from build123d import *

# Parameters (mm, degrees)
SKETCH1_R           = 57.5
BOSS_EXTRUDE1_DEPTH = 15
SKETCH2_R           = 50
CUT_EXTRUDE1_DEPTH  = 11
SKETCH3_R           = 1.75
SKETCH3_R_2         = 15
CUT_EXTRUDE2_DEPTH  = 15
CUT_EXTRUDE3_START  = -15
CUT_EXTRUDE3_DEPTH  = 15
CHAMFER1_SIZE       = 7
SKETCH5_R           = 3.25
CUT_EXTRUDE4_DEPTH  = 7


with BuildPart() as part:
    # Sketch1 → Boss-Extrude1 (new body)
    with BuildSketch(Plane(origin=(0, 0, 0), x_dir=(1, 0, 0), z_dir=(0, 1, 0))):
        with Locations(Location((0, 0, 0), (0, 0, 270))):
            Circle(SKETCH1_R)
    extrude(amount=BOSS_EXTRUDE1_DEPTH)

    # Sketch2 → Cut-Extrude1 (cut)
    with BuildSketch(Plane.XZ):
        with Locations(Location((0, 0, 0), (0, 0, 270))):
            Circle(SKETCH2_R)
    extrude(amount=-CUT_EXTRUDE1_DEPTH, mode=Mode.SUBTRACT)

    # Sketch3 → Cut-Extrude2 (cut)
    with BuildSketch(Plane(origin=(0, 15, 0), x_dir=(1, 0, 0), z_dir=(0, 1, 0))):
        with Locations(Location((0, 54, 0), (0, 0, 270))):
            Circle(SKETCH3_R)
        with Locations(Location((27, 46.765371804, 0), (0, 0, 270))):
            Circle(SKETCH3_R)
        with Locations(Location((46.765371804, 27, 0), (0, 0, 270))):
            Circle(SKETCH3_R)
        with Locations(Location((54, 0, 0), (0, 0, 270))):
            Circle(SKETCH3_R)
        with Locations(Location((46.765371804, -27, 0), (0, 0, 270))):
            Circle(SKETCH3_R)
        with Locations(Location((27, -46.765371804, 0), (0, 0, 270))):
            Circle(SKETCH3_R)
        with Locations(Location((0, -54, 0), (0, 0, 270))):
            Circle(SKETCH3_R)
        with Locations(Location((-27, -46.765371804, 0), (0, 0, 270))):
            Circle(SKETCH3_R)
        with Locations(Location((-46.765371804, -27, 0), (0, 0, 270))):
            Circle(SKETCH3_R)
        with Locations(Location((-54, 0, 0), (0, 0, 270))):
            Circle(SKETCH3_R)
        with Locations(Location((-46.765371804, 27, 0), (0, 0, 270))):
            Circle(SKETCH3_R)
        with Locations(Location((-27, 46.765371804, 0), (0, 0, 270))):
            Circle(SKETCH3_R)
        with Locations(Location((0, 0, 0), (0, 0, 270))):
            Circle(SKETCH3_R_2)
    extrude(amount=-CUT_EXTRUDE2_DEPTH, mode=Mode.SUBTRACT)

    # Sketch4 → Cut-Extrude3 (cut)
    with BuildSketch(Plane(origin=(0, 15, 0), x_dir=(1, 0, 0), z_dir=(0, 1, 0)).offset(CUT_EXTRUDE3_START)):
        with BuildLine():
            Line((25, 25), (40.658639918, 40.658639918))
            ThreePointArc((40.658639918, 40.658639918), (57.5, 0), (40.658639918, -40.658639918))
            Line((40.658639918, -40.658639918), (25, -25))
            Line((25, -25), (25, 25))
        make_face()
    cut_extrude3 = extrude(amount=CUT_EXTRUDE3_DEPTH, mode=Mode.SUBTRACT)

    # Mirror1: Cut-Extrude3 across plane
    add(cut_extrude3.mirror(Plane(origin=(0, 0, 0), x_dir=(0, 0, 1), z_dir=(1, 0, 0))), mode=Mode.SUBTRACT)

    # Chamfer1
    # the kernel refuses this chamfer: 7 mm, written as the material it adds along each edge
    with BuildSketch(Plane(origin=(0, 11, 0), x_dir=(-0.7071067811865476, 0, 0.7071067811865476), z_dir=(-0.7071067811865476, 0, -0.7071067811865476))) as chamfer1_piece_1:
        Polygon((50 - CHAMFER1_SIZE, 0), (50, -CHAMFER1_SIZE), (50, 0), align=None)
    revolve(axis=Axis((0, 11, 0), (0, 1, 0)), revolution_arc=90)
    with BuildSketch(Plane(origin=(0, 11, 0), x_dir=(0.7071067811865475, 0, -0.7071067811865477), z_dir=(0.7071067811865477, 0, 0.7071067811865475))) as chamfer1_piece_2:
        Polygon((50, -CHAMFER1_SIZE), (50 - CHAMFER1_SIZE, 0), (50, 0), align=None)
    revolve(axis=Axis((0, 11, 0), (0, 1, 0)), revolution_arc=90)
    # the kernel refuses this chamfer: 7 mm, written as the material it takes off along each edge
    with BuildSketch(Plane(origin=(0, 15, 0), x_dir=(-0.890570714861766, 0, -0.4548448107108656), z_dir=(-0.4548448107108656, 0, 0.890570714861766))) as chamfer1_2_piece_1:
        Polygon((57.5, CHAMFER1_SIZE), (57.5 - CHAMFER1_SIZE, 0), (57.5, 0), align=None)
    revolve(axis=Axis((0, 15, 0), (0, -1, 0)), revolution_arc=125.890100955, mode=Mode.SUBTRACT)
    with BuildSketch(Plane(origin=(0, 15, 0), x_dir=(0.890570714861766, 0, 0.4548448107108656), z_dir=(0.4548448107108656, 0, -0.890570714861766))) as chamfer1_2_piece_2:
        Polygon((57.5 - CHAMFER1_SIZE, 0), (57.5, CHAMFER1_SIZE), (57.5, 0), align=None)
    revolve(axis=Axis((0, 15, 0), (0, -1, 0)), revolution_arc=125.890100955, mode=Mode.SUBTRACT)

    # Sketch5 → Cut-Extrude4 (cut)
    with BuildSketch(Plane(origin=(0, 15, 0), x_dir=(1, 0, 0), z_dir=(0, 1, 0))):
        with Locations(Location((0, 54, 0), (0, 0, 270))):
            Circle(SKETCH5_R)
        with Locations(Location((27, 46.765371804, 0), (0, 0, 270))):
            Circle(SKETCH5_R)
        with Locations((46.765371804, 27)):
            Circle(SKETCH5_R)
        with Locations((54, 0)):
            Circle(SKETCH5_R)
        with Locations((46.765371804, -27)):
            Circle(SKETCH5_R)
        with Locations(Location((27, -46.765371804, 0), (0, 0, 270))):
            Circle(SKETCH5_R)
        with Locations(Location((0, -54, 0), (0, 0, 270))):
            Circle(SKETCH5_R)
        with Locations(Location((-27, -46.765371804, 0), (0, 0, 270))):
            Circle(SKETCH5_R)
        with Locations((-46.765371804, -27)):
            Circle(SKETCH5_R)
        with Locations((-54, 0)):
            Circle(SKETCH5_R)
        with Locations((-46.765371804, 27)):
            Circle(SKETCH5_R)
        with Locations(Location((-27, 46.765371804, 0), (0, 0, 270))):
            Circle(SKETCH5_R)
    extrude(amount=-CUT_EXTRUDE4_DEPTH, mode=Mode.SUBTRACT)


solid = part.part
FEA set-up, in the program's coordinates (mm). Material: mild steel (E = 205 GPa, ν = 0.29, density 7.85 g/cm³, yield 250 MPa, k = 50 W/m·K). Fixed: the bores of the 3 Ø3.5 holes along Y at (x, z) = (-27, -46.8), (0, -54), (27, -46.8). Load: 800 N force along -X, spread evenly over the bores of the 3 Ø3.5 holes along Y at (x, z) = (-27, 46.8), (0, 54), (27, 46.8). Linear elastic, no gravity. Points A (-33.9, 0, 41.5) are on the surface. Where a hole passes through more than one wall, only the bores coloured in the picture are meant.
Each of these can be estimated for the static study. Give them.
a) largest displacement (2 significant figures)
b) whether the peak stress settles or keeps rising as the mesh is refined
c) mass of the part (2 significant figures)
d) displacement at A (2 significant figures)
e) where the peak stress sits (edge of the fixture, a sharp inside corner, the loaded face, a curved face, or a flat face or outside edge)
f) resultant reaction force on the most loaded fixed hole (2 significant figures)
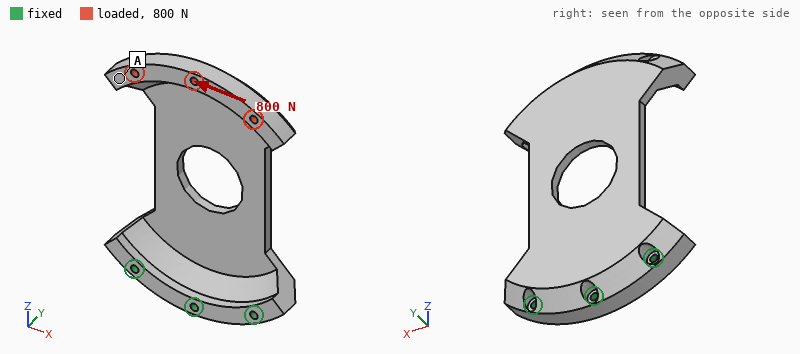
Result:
0.32 mm
keeps rising
280 g
0.28 mm
edge of the fixture
1.4 kN
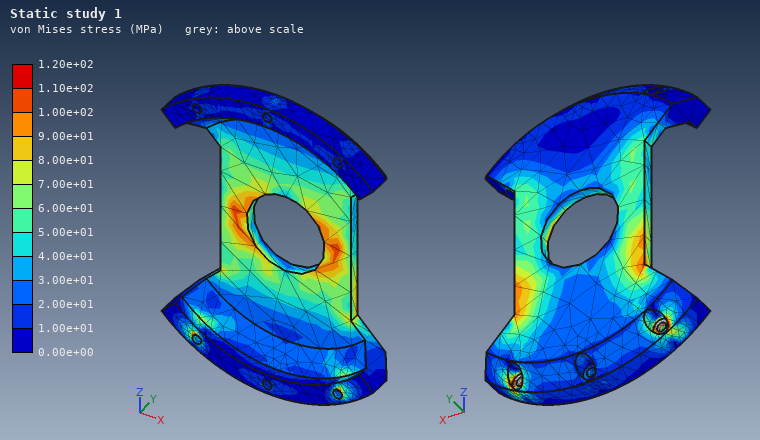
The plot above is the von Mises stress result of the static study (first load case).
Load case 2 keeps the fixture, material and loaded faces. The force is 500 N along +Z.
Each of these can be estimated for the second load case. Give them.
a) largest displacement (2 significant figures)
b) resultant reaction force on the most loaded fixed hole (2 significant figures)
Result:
0.55 mm
200 N
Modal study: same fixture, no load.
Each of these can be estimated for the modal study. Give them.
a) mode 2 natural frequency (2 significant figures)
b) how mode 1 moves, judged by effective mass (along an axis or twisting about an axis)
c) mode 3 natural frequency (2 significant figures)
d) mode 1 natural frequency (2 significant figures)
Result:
720 Hz
along Y
1800 Hz
210 Hz
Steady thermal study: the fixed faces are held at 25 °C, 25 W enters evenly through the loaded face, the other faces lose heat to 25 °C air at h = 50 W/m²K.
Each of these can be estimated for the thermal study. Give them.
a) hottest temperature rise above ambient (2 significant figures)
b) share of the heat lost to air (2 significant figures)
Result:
72 K
90 %
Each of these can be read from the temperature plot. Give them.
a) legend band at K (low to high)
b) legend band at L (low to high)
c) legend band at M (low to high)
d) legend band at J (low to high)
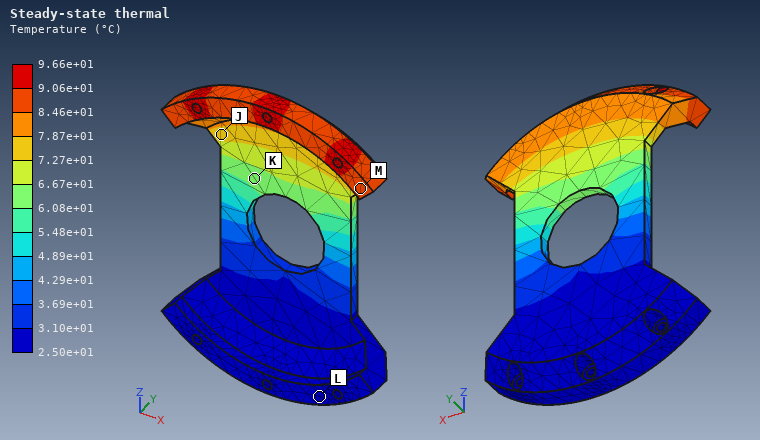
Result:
6.08e+01 to 6.67e+01 °C
2.50e+01 to 3.10e+01 °C
8.46e+01 to 9.06e+01 °C
7.27e+01 to 7.87e+01 °C
